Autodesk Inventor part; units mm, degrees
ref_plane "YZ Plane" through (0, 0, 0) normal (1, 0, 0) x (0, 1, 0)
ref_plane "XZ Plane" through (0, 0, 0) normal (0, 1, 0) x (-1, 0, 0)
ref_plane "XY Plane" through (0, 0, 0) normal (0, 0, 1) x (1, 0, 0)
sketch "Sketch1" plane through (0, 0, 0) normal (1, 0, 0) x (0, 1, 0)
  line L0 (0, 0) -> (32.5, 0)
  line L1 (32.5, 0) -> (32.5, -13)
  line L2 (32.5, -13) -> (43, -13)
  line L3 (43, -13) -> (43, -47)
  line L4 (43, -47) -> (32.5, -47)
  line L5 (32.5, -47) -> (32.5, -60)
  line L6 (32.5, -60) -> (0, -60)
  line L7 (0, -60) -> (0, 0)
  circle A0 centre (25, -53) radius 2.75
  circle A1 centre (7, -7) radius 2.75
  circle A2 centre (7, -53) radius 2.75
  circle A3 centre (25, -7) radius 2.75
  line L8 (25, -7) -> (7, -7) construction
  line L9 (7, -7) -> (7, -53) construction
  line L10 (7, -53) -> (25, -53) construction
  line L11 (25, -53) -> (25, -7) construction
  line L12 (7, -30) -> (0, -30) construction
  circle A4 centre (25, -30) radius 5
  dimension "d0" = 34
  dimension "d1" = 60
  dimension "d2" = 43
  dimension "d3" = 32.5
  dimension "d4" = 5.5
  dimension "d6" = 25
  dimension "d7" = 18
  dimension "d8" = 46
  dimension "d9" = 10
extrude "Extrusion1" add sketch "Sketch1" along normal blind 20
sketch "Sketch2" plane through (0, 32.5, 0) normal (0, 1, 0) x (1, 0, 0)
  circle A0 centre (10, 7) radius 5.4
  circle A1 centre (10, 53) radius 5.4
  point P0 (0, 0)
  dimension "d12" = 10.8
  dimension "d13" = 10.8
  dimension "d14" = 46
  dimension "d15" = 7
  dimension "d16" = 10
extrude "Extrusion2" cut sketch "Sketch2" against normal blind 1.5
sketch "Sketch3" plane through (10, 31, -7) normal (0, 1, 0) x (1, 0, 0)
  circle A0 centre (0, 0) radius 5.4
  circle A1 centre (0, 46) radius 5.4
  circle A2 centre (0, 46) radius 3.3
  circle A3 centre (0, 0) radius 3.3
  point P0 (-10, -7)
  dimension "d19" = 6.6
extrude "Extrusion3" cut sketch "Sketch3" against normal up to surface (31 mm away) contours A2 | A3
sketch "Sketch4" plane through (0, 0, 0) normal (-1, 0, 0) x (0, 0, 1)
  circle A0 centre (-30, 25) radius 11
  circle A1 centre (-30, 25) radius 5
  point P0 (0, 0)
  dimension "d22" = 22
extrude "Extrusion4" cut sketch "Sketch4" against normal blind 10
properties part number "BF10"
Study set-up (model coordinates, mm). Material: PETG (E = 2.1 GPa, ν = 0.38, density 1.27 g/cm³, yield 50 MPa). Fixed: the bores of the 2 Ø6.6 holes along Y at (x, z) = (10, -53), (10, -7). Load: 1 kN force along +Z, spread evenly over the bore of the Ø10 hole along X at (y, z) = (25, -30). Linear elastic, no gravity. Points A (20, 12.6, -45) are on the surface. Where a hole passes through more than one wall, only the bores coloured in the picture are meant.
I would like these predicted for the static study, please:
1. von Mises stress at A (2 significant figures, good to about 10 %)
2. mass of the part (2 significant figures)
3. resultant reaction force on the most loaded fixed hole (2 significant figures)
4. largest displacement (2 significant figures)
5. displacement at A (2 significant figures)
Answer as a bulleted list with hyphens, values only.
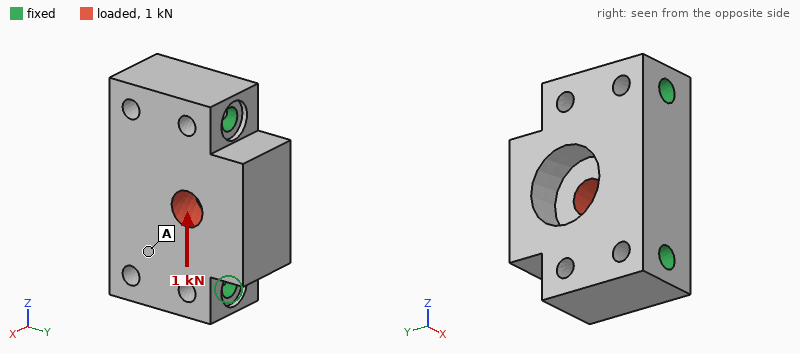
- 0.76 MPa
- 48 g
- 520 N
- 29 µm
- 5.9 µm
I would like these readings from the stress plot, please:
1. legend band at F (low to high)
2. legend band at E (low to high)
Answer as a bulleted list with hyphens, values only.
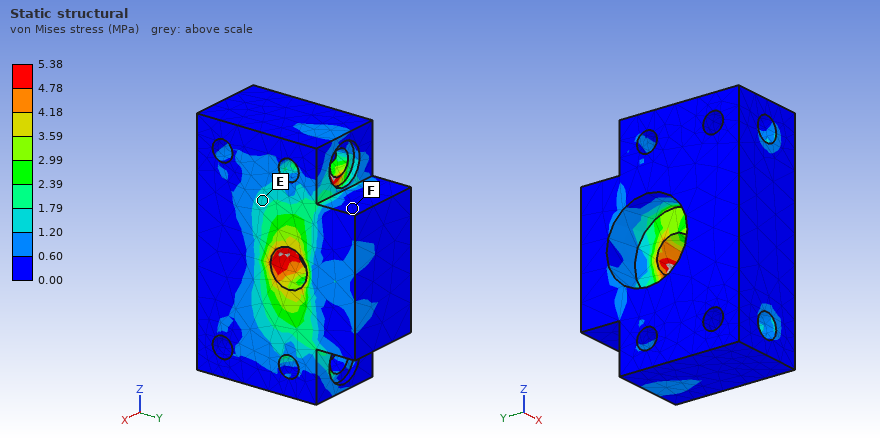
- 0.00 to 0.60 MPa
- 1.20 to 1.79 MPa
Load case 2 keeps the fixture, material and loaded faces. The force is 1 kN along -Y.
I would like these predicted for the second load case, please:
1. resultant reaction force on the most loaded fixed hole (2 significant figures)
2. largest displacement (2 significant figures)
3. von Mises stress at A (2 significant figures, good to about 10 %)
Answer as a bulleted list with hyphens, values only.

- 510 N
- 52 µm
- 2.1 MPa
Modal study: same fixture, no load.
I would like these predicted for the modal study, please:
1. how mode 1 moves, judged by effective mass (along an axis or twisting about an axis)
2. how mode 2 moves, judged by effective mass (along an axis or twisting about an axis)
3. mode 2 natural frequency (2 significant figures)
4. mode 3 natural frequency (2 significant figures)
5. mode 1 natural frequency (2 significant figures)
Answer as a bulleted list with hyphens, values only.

- along X
- along X
- 6300 Hz
- 7200 Hz
- 4000 Hz
